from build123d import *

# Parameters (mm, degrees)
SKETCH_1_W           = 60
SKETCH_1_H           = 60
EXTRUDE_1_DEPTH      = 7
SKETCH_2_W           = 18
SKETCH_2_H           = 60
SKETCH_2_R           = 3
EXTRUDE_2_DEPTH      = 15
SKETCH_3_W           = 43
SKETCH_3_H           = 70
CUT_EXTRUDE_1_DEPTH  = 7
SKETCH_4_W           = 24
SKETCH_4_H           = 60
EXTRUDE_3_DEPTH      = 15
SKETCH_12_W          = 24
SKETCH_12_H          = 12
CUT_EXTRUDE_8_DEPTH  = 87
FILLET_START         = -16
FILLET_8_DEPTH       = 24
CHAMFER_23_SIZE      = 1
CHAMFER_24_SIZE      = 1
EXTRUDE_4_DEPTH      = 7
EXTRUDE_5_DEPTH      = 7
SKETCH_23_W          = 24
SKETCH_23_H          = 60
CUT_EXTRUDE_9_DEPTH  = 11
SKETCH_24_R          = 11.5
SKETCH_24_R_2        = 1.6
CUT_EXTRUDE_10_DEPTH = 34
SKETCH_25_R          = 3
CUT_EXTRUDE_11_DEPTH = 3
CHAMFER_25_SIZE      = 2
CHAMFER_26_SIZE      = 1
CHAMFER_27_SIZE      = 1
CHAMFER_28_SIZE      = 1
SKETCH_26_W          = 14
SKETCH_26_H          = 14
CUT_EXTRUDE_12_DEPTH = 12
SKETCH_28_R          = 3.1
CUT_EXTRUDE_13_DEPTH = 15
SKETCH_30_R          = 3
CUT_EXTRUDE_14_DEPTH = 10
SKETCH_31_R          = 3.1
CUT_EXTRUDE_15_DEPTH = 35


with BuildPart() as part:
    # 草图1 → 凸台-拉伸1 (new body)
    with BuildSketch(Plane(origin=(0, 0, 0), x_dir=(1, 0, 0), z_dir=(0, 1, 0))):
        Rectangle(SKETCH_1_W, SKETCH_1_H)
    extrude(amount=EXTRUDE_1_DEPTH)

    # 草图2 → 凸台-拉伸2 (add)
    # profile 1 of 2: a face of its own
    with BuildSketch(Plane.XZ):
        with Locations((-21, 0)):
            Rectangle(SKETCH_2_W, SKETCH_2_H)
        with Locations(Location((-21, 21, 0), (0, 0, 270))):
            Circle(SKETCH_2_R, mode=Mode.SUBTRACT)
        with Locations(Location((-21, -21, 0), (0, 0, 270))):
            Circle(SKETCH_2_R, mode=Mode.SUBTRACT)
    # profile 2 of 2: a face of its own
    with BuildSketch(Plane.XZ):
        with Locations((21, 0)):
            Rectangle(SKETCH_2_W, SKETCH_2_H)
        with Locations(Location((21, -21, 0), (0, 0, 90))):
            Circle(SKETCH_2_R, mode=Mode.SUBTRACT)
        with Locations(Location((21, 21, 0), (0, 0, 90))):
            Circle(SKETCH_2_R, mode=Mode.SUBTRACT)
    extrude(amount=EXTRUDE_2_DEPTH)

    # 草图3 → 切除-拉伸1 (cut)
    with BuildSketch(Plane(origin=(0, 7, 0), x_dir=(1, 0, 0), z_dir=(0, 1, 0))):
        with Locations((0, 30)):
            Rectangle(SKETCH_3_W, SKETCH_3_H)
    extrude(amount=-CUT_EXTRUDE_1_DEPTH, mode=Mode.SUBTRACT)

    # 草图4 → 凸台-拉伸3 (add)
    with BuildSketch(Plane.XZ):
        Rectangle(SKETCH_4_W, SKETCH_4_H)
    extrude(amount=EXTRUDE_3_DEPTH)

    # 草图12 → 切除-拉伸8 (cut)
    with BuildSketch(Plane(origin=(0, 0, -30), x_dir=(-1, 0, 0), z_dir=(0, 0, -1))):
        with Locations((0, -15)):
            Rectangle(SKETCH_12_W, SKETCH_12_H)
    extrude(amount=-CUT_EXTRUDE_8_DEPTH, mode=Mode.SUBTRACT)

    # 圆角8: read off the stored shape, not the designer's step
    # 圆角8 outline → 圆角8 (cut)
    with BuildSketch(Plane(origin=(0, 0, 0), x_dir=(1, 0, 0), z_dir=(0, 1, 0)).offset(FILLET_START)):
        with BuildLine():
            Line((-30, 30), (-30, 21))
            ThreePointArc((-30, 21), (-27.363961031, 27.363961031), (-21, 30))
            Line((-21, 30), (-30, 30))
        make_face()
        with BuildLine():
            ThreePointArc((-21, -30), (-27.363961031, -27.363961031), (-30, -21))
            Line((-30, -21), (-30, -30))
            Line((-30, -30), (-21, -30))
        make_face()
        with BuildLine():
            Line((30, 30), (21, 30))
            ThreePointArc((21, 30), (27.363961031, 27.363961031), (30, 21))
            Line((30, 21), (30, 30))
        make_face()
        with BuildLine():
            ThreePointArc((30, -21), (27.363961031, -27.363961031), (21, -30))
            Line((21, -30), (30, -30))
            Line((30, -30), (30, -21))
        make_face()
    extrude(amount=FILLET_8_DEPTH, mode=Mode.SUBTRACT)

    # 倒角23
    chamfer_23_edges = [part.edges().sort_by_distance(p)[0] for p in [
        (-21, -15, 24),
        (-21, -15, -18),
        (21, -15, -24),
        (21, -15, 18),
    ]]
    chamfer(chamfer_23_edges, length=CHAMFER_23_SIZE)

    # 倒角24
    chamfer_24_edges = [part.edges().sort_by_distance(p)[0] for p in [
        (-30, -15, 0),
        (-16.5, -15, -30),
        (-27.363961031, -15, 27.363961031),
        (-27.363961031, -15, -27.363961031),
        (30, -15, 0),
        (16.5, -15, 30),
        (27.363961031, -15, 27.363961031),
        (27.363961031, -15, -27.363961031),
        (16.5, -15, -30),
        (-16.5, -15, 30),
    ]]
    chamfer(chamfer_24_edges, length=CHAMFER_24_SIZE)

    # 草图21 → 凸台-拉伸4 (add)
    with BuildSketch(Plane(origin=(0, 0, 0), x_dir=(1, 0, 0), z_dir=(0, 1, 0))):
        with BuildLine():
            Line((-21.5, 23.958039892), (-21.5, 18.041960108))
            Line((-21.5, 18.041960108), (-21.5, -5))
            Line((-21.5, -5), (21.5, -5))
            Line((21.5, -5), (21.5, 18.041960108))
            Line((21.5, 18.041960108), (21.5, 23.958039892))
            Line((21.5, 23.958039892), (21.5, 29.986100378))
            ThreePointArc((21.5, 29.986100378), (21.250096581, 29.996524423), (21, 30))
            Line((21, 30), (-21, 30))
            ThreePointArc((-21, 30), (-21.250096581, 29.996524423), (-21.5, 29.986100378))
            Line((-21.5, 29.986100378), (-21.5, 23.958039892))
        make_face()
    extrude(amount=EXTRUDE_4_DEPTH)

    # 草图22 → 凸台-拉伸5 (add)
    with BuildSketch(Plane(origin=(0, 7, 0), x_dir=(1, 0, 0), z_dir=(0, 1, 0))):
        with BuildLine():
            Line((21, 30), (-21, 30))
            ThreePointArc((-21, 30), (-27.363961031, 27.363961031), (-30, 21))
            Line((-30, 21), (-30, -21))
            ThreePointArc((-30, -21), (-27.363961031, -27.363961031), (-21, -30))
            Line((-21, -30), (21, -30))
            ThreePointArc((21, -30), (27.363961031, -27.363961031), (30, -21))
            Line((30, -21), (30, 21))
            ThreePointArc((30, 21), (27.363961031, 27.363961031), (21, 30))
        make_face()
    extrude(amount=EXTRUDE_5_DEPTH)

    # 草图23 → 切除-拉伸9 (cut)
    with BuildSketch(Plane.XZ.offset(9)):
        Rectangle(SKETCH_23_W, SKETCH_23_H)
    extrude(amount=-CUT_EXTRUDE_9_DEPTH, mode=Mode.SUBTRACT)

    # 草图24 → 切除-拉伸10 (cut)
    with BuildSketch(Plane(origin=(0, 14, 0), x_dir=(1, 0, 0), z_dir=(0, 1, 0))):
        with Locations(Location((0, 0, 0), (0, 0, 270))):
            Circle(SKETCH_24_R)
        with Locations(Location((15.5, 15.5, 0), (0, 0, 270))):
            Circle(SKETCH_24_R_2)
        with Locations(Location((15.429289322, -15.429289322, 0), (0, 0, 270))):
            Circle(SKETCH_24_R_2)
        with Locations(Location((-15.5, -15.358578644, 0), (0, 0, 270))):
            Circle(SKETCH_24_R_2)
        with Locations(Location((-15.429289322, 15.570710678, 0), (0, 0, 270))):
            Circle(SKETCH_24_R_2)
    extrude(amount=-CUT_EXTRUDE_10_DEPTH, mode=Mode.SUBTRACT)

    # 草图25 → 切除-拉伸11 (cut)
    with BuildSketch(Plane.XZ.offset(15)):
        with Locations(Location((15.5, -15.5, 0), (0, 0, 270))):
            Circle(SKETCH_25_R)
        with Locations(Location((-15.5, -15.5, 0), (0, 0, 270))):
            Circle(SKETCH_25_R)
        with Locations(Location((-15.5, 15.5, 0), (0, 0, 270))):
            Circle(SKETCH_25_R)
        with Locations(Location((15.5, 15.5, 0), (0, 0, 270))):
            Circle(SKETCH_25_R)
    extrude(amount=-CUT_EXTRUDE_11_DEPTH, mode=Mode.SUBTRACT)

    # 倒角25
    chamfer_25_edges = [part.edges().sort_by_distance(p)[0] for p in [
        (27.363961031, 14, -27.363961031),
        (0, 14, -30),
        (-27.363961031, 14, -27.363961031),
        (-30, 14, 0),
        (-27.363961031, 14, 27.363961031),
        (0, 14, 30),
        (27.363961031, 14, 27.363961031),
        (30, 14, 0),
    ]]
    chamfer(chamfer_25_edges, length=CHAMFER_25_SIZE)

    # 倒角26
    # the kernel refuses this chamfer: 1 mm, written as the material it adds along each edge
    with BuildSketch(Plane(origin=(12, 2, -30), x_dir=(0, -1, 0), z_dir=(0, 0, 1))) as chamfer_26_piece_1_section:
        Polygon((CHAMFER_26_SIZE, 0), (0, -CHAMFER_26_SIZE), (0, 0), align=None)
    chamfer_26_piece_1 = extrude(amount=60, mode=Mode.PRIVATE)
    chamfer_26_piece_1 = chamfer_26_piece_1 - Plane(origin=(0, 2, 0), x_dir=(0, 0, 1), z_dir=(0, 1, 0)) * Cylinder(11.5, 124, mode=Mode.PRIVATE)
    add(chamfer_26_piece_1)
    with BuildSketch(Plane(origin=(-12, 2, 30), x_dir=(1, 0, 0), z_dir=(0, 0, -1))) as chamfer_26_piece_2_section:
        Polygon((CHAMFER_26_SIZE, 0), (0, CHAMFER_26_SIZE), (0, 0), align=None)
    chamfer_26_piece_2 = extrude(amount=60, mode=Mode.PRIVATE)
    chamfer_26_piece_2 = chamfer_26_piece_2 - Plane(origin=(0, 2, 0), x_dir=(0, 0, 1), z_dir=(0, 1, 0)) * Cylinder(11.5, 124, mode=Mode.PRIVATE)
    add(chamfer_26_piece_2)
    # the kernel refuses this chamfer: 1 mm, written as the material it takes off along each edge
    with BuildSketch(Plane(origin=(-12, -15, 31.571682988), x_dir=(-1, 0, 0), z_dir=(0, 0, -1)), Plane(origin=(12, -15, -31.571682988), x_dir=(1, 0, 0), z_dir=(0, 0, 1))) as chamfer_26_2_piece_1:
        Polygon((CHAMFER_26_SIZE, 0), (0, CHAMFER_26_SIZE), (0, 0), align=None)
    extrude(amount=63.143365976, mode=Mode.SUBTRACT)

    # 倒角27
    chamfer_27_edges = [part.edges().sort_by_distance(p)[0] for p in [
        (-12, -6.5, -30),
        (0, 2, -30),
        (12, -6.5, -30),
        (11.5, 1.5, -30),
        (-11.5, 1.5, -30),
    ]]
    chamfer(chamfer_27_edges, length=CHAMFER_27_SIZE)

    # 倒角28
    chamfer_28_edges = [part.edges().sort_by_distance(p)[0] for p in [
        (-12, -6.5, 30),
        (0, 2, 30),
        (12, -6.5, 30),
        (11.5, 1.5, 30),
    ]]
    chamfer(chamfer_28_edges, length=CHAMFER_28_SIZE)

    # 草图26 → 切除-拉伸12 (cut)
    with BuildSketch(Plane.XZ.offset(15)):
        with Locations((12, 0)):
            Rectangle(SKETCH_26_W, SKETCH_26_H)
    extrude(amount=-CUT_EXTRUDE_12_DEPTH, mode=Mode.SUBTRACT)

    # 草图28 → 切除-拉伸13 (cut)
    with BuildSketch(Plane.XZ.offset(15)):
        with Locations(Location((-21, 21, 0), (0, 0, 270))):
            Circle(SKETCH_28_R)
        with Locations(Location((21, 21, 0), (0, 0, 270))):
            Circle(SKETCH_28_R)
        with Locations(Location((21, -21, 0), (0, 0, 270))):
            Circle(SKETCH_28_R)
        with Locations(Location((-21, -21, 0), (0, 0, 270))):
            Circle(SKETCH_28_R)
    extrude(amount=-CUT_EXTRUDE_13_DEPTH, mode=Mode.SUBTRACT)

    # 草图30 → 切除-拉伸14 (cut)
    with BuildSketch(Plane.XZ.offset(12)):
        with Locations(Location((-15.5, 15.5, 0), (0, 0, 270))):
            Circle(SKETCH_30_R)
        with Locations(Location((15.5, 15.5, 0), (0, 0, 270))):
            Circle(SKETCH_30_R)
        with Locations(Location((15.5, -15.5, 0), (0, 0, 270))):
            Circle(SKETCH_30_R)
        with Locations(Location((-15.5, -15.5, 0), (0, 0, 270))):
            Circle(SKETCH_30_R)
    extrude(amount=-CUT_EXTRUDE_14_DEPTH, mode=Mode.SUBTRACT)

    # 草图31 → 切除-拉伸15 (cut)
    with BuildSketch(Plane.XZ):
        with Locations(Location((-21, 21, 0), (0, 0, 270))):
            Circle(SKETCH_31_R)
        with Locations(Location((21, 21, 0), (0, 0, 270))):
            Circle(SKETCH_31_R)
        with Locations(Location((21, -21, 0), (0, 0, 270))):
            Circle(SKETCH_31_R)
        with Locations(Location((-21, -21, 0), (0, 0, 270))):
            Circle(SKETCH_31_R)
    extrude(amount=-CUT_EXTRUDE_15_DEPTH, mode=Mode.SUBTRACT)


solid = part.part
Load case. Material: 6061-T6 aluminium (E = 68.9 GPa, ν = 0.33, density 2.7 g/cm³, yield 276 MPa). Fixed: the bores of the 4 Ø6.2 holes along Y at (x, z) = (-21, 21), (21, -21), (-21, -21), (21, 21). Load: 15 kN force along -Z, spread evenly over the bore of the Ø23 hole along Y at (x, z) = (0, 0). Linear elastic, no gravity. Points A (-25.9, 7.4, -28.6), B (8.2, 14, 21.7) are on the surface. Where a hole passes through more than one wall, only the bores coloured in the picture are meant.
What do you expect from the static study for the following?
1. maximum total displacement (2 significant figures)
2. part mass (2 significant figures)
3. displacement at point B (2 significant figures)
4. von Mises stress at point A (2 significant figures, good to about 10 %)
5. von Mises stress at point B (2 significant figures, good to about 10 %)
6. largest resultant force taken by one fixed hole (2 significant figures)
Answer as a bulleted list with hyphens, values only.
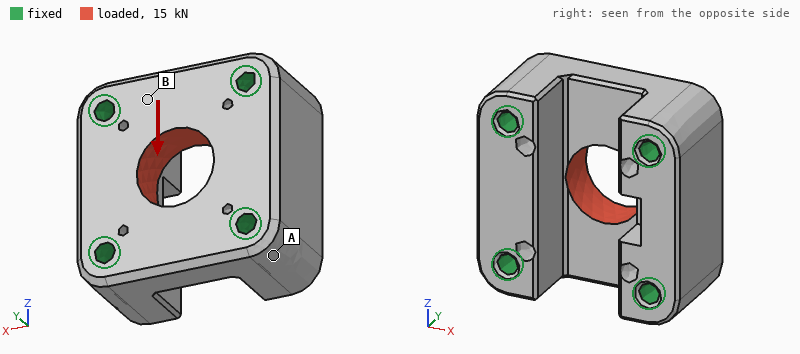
- 8.5 µm
- 180 g
- 5.2 µm
- 5.2 MPa
- 12 MPa
- 4.1 kN
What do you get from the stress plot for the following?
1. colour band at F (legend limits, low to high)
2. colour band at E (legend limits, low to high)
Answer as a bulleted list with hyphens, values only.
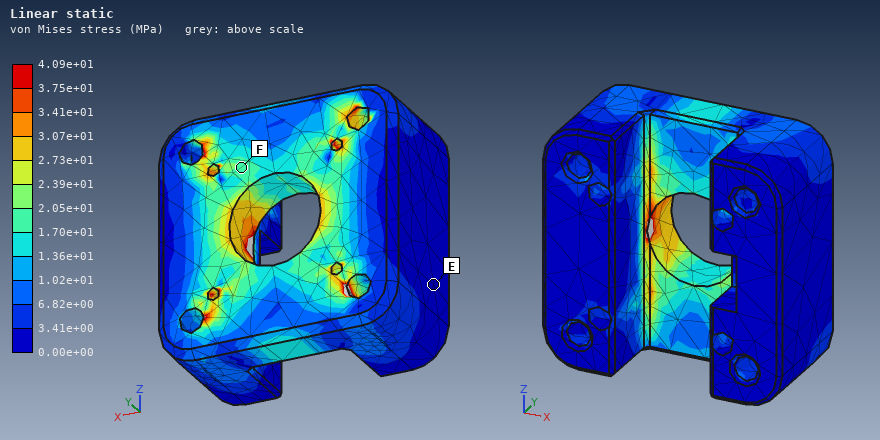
- 1.70e+01 to 2.05e+01 MPa
- 0.00e+00 to 3.41e+00 MPa
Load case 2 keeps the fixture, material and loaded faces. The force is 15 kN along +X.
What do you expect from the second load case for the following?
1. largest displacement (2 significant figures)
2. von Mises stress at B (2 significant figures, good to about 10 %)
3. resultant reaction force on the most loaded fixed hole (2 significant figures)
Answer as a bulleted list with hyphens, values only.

- 9.6 µm
- 6.6 MPa
- 4.0 kN
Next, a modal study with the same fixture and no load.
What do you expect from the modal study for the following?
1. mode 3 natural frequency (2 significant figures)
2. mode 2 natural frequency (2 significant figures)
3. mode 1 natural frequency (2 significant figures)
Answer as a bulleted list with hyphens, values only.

- 29 kHz
- 28 kHz
- 26 kHz
